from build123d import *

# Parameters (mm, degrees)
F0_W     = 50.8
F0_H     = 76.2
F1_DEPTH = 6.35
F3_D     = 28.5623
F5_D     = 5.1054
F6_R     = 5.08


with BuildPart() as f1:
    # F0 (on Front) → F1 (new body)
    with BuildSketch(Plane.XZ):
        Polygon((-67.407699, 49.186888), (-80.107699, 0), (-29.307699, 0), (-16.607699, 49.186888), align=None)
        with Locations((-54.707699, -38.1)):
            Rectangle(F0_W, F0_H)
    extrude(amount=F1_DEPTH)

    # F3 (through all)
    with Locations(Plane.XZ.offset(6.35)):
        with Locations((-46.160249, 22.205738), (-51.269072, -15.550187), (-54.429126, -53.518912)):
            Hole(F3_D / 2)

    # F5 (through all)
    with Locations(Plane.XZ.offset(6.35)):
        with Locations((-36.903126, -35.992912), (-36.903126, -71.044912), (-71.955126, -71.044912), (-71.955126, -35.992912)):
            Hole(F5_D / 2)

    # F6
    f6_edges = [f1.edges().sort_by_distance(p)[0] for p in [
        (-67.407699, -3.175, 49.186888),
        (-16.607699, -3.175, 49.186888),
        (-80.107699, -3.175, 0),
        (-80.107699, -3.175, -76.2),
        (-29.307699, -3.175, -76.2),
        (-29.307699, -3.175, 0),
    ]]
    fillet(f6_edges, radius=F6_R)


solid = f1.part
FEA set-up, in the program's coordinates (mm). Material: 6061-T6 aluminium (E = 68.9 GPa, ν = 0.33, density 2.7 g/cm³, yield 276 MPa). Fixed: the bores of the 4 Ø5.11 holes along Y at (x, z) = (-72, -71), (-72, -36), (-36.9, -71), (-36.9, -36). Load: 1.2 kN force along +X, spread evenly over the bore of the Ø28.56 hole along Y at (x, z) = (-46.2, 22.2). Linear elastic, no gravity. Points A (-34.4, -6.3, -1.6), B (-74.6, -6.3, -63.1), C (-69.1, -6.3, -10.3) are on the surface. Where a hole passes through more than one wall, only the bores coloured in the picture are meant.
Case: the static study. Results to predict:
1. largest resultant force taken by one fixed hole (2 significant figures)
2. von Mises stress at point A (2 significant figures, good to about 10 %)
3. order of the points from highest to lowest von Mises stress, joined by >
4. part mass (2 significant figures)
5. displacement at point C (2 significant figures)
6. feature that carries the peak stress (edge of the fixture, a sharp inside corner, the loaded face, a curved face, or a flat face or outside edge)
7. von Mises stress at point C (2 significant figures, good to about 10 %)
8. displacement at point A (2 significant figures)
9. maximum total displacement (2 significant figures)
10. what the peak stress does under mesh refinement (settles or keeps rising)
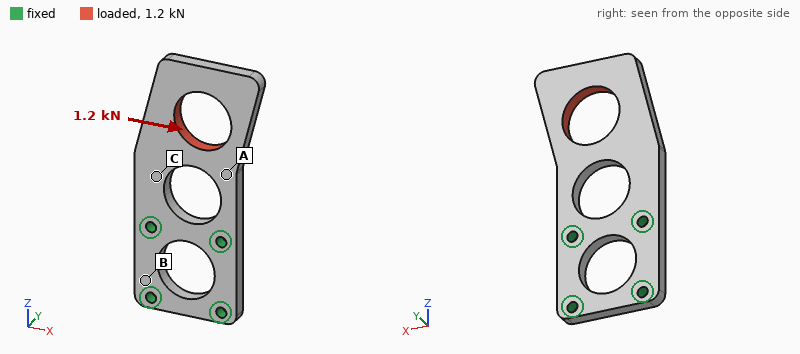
1.6 kN
12 MPa
C > A > B
74 g
0.030 mm
edge of the fixture
20 MPa
0.047 mm
0.10 mm
keeps rising
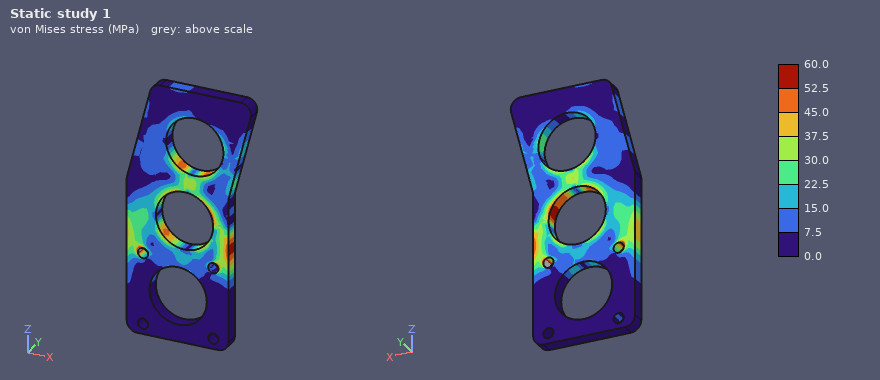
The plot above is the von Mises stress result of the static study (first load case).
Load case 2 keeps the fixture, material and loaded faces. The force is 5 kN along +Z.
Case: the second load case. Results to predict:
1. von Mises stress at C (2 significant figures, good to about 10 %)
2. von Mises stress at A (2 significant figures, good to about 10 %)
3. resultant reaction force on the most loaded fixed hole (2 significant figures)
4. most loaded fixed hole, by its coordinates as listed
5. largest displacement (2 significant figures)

25 MPa
41 MPa
3.3 kN
(-36.9, -36)
91 µm
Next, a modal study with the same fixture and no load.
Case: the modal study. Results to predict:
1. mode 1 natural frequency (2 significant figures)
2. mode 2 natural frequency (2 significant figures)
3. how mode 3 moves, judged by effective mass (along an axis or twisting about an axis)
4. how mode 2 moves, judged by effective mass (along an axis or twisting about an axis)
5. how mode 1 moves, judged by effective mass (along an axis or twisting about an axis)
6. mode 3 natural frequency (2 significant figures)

600 Hz
2000 Hz
along X
twisting about Z
along Y
3200 Hz
